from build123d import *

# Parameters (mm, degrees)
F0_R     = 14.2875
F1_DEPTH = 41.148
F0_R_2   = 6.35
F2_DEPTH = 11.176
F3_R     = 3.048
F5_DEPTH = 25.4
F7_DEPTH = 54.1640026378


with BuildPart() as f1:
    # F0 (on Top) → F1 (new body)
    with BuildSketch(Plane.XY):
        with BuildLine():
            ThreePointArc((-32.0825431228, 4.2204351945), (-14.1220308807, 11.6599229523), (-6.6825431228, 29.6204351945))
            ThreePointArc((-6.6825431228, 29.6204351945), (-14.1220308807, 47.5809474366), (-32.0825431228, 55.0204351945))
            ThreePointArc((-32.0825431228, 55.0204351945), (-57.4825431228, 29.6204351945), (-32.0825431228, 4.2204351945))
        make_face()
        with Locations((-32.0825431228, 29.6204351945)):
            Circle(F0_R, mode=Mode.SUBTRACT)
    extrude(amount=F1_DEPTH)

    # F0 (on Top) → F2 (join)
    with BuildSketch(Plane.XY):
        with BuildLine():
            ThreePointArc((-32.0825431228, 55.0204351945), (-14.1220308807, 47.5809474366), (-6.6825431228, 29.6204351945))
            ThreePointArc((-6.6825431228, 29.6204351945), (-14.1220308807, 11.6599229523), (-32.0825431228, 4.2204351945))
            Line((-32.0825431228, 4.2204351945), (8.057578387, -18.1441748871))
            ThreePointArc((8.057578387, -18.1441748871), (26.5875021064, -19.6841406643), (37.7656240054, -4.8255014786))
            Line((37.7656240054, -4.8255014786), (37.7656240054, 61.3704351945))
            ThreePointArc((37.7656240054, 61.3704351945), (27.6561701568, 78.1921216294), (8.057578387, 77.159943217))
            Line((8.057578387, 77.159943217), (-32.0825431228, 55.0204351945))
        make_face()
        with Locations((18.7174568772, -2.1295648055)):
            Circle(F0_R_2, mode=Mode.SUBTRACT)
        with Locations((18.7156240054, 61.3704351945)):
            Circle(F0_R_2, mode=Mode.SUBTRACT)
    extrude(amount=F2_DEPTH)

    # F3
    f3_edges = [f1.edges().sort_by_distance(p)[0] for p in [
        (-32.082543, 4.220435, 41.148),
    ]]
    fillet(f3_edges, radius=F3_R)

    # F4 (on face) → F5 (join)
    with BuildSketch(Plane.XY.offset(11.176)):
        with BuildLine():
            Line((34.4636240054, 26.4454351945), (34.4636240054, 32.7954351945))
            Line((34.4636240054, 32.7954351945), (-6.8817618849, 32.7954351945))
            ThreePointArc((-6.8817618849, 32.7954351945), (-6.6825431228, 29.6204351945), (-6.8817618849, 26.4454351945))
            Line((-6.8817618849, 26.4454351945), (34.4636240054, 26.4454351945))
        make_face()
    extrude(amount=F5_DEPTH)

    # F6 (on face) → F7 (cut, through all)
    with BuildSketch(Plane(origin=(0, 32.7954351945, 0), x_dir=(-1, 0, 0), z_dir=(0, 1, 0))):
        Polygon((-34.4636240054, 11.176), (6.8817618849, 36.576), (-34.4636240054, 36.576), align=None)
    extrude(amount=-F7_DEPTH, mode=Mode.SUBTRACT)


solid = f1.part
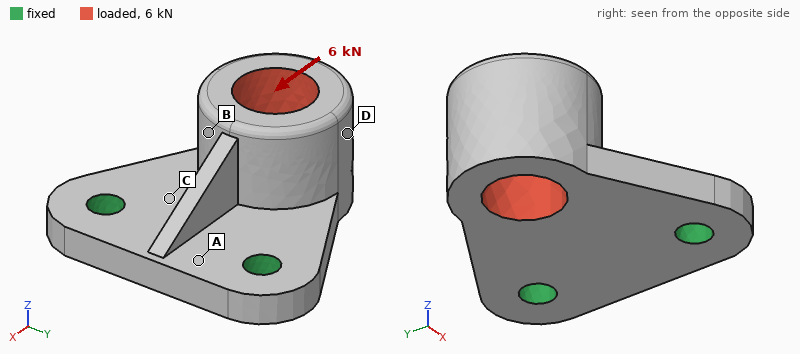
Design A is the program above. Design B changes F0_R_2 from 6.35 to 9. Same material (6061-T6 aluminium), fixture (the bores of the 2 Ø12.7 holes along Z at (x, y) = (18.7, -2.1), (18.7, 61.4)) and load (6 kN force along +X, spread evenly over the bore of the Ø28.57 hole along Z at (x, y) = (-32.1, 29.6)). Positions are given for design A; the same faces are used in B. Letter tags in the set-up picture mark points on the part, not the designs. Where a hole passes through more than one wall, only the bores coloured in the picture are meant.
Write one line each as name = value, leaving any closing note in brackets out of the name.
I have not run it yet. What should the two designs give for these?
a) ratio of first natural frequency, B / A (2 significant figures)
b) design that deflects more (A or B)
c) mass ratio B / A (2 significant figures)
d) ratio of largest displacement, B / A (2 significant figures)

ratio of first natural frequency, B / A = 1.1
design that deflects more = A
mass ratio B / A = 0.97
ratio of largest displacement, B / A = 0.84
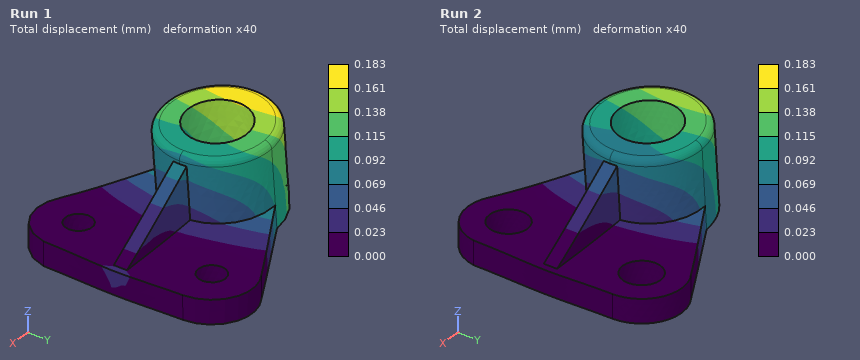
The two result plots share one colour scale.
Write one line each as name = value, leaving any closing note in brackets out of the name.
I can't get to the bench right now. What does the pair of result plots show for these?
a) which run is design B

which run is design B = Run 2
